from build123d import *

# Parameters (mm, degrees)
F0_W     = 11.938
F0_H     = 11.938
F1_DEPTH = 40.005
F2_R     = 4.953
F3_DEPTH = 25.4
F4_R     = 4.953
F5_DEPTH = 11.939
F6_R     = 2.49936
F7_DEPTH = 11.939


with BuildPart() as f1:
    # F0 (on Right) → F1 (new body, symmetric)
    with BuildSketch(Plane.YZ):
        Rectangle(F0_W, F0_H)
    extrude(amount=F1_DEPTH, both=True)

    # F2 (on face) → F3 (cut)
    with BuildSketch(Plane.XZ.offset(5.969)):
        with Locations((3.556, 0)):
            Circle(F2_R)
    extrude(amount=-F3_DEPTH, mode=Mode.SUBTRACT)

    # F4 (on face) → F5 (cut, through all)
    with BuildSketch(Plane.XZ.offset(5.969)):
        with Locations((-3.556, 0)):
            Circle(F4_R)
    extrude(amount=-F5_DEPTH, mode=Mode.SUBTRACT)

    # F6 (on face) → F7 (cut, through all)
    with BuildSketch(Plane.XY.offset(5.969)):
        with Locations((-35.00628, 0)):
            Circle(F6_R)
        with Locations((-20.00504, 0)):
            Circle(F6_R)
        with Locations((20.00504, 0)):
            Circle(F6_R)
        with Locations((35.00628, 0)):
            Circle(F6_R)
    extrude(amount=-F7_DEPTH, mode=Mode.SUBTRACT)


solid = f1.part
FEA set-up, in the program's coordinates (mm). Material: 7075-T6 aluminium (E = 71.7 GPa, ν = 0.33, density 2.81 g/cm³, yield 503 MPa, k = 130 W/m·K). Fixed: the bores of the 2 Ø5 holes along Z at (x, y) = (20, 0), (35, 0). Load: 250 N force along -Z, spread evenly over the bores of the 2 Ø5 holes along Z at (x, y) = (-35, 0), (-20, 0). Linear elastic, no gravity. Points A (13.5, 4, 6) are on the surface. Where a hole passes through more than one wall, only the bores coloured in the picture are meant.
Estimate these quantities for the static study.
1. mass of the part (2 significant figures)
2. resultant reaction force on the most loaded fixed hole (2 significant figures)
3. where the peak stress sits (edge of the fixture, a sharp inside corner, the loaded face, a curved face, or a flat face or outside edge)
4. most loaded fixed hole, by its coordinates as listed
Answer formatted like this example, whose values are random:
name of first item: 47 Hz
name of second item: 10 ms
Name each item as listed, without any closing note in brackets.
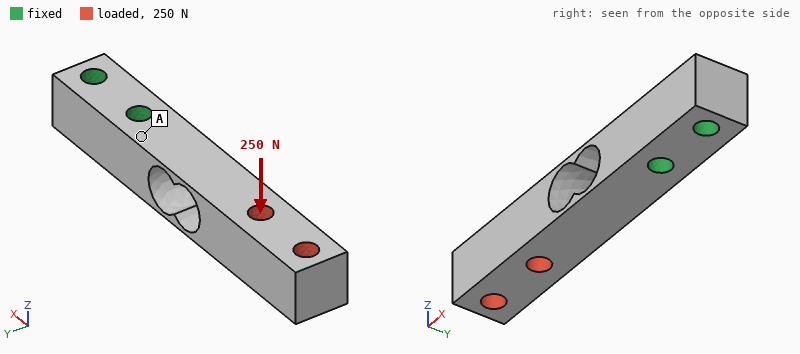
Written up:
mass of the part: 25 g
resultant reaction force on the most loaded fixed hole: 310 N
where the peak stress sits: a curved face
most loaded fixed hole, by its coordinates as listed: (20, 0)
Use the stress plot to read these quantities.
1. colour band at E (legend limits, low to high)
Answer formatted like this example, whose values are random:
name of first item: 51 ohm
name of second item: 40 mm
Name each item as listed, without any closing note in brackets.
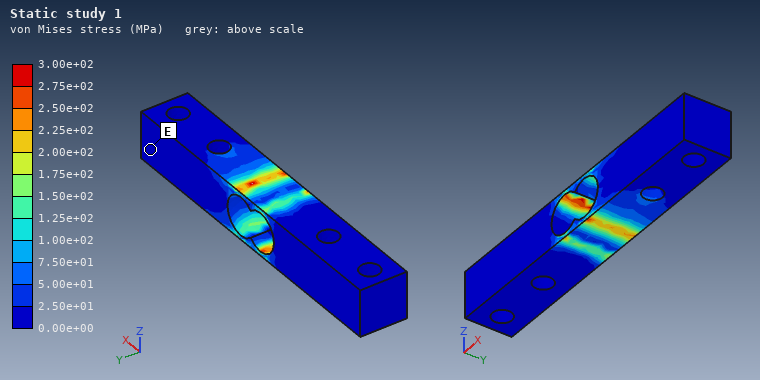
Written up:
colour band at E: 0.00e+00 to 2.50e+01 MPa
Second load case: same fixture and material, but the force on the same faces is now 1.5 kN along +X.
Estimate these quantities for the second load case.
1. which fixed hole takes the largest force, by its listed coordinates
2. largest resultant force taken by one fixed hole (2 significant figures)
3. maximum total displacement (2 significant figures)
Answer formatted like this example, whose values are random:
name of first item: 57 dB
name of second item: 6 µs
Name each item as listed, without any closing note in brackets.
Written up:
which fixed hole takes the largest force, by its listed coordinates: (20, 0)
largest resultant force taken by one fixed hole: 1.4 kN
maximum total displacement: 20 µm
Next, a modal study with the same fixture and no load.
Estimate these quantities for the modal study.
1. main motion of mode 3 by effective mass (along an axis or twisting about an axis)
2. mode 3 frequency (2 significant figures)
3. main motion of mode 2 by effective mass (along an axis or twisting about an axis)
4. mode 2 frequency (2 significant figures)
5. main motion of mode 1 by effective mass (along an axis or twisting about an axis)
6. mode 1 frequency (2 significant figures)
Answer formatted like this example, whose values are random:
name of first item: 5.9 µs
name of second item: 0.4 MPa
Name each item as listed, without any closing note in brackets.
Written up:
main motion of mode 3 by effective mass: twisting about X
mode 3 frequency: 6700 Hz
main motion of mode 2 by effective mass: along Y
mode 2 frequency: 1700 Hz
main motion of mode 1 by effective mass: along Z
mode 1 frequency: 1400 Hz
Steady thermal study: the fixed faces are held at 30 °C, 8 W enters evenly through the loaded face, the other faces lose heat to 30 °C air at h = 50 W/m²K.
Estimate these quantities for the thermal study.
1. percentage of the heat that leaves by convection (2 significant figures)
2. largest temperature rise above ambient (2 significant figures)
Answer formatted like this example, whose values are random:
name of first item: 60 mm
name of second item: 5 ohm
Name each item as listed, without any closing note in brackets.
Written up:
percentage of the heat that leaves by convection: 37 %
largest temperature rise above ambient: 31 K
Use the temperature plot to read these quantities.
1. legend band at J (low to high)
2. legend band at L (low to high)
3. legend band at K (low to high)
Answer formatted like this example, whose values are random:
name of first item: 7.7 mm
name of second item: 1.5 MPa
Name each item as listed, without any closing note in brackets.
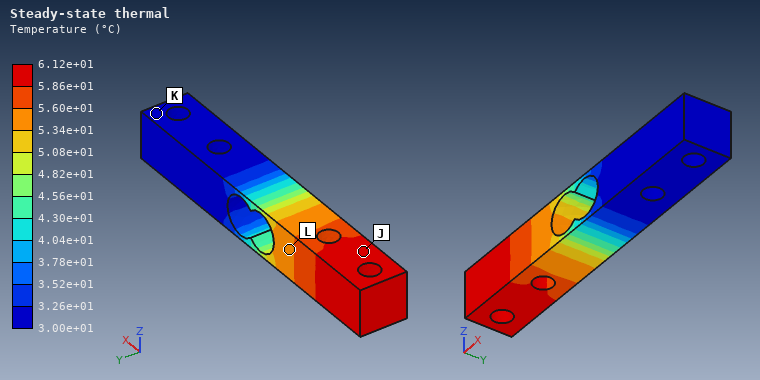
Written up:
legend band at J: 5.86e+01 to 6.12e+01 °C
legend band at L: 5.34e+01 to 5.60e+01 °C
legend band at K: 3.00e+01 to 3.26e+01 °C
